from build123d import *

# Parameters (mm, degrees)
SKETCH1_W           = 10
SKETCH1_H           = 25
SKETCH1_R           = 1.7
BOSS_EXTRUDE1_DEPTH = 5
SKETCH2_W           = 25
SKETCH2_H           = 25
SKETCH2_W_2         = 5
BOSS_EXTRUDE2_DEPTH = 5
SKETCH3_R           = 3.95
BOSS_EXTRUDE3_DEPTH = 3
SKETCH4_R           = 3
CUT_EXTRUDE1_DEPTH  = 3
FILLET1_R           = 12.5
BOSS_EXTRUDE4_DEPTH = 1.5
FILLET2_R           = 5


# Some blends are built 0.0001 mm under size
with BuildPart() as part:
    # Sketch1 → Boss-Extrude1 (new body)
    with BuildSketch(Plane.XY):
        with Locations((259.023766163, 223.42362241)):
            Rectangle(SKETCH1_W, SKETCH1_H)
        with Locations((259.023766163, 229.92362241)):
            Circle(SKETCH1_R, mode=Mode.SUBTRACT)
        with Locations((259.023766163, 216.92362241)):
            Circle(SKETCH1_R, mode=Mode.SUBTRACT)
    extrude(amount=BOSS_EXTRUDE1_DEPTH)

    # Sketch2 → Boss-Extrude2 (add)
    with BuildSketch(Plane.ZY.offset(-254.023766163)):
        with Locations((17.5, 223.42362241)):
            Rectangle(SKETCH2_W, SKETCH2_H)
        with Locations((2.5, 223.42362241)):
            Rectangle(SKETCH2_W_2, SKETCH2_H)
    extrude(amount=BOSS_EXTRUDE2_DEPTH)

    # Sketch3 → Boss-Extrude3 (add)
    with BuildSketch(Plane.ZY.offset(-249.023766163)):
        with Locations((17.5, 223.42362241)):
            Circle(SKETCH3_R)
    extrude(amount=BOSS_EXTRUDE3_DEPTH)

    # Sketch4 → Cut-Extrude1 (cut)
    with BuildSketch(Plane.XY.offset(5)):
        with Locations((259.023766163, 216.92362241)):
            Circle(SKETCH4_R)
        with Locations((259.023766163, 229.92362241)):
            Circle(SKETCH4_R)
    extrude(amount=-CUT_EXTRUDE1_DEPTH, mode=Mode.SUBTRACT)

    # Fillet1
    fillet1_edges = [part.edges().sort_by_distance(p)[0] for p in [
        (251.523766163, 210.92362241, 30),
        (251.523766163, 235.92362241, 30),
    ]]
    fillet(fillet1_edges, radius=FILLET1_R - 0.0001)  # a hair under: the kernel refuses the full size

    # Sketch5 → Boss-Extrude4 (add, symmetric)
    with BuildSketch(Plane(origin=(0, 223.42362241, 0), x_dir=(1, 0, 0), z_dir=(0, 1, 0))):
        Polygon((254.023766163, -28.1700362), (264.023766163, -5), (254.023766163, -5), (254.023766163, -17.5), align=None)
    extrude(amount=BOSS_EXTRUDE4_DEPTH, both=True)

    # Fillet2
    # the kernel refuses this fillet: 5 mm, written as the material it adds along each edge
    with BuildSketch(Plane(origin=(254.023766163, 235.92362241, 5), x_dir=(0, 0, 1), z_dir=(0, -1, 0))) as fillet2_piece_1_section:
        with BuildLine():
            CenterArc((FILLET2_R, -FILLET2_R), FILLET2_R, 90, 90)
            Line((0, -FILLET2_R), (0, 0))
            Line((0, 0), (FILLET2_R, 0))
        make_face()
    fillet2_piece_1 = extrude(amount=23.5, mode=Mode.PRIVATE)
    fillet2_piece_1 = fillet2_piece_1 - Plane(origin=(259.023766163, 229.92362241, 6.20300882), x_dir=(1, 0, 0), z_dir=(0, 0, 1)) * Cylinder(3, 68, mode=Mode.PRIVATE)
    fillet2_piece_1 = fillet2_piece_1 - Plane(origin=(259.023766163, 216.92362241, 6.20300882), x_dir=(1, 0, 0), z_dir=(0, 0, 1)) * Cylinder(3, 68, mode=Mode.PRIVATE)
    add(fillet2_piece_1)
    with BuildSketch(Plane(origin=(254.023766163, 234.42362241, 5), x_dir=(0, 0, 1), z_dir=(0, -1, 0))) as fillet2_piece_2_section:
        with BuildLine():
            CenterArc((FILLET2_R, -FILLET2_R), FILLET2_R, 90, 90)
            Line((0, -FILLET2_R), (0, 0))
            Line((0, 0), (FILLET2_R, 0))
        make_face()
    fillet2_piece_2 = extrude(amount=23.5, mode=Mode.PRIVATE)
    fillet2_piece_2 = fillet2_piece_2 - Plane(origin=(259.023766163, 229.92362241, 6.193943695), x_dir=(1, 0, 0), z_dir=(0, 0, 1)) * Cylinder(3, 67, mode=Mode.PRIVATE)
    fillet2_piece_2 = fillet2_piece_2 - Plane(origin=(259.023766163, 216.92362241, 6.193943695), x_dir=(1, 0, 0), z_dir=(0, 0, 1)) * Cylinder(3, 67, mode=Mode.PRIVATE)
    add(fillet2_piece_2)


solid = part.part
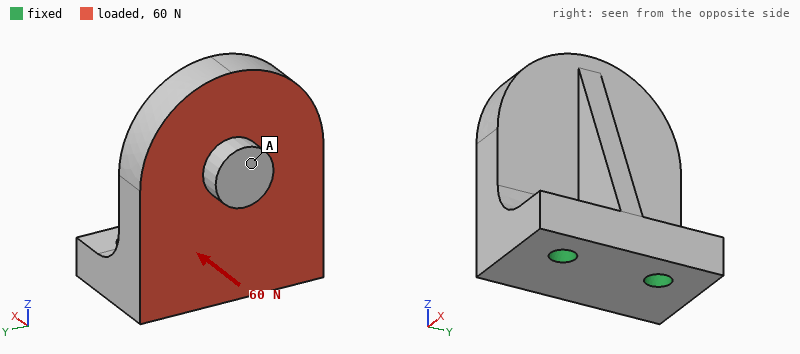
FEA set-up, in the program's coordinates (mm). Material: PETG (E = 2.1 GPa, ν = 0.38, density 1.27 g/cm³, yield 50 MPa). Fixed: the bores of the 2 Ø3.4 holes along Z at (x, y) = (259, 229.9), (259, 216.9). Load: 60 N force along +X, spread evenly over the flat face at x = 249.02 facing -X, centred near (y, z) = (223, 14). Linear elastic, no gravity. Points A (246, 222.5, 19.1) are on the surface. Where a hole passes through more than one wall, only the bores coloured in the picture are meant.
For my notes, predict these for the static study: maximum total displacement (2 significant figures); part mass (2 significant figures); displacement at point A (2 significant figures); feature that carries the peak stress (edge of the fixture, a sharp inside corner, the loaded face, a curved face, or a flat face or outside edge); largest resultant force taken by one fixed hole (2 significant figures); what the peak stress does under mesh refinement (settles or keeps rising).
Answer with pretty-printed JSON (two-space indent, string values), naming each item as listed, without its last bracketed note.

{
  "maximum total displacement": "0.49 mm",
  "part mass": "6.4 g",
  "displacement at point A": "0.35 mm",
  "feature that carries the peak stress": "edge of the fixture",
  "largest resultant force taken by one fixed hole": "31 N",
  "what the peak stress does under mesh refinement": "keeps rising"
}
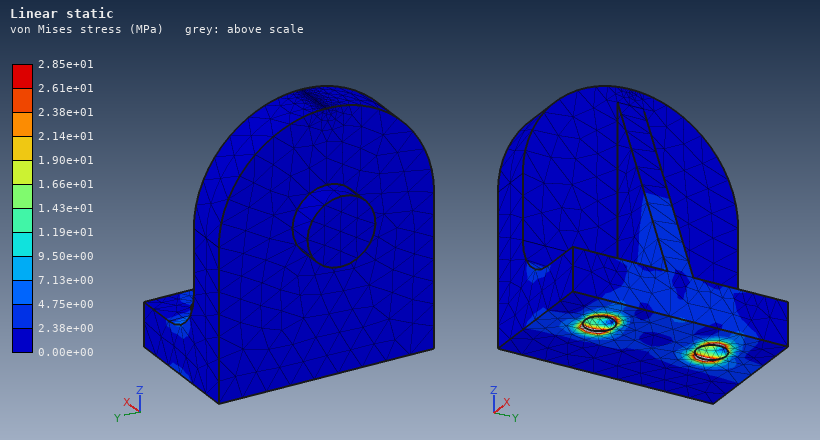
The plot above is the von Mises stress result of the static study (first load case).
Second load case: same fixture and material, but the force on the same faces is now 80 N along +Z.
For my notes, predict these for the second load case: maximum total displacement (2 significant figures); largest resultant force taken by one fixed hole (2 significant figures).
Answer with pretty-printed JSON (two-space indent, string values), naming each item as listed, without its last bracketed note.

{
  "maximum total displacement": "0.47 mm",
  "largest resultant force taken by one fixed hole": "40 N"
}
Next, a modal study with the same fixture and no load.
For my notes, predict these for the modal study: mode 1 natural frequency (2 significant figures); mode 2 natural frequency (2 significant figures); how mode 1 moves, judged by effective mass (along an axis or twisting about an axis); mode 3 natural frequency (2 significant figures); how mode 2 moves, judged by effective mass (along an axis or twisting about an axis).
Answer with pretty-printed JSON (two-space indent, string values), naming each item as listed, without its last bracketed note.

{
  "mode 1 natural frequency": "930 Hz",
  "mode 2 natural frequency": "2100 Hz",
  "how mode 1 moves, judged by effective mass": "along X",
  "mode 3 natural frequency": "4000 Hz",
  "how mode 2 moves, judged by effective mass": "along Y"
}
